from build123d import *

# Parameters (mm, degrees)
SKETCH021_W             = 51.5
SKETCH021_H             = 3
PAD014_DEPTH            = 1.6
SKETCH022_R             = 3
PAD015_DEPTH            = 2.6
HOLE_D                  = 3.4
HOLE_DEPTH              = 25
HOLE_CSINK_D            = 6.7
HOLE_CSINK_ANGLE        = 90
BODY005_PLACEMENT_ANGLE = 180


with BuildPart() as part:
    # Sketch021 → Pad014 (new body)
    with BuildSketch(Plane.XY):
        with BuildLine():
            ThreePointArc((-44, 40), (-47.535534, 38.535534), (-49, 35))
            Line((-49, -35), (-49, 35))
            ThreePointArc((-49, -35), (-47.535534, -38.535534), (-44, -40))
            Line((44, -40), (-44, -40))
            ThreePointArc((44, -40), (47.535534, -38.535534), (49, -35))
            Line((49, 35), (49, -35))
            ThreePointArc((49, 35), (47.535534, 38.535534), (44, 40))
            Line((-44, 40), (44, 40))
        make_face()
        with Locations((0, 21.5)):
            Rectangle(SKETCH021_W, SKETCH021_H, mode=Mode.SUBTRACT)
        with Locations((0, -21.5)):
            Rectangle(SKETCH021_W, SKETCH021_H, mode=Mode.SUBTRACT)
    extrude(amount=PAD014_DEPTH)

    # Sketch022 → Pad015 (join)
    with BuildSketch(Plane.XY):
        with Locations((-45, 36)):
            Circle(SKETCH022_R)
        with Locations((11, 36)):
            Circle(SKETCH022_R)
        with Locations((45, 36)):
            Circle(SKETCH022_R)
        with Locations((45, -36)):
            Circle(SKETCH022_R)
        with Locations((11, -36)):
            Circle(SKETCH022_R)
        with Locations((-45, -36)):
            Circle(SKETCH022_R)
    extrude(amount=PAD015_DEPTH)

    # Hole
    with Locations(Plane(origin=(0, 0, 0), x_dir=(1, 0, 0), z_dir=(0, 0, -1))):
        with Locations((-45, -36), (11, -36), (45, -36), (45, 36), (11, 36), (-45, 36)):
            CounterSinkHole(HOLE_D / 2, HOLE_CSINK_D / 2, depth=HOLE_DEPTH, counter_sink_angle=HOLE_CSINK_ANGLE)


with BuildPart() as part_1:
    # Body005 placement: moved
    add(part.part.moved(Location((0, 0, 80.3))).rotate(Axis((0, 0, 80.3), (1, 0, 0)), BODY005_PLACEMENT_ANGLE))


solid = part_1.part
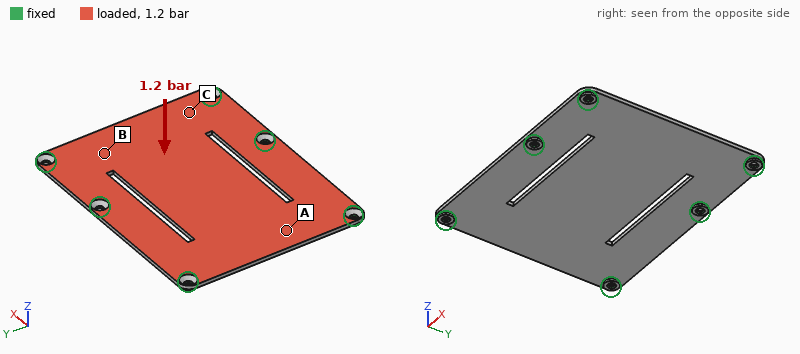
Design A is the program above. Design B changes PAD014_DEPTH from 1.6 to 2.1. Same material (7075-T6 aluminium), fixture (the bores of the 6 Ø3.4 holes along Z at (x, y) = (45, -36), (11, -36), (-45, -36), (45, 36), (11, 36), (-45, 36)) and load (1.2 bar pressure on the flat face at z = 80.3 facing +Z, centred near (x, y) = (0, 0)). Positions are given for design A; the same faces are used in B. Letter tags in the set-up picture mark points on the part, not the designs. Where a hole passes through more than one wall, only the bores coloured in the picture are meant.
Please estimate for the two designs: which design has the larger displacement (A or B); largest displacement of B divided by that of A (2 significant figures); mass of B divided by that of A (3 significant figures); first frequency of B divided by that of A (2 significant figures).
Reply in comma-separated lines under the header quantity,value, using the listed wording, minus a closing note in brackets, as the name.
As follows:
quantity,value
which design has the larger displacement,A
largest displacement of B divided by that of A,0.49
mass of B divided by that of A,1.31
first frequency of B divided by that of A,1.3
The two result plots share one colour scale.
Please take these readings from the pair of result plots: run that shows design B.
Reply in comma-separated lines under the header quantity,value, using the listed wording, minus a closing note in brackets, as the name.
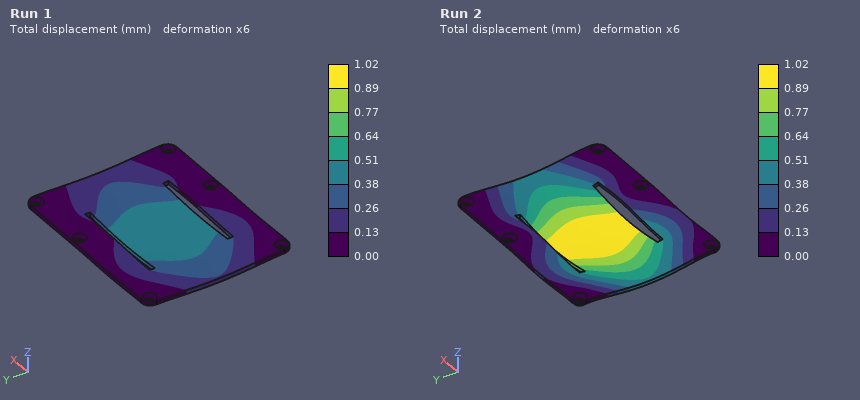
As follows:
quantity,value
run that shows design B,Run 1
